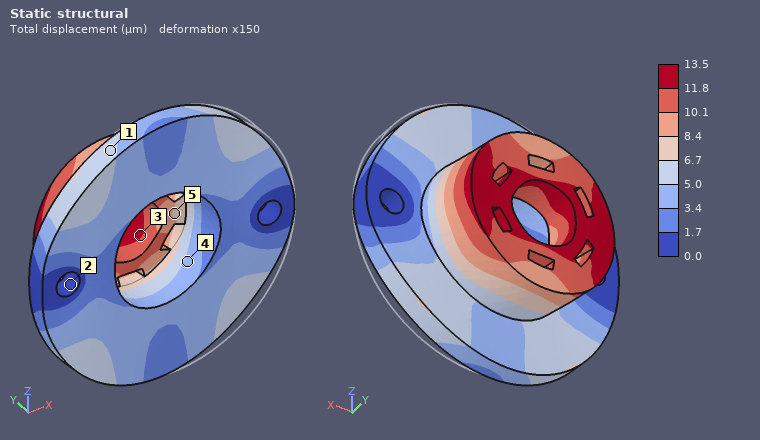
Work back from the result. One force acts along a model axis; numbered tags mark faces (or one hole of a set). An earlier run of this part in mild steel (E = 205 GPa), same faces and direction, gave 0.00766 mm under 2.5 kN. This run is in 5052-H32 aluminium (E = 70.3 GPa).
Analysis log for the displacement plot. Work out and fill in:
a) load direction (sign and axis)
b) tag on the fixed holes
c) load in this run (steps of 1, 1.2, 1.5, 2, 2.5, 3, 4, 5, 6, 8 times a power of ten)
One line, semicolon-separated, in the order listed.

-X; 2; 1.5 kN
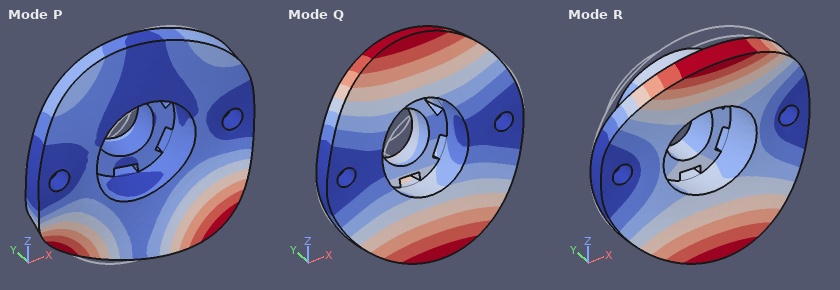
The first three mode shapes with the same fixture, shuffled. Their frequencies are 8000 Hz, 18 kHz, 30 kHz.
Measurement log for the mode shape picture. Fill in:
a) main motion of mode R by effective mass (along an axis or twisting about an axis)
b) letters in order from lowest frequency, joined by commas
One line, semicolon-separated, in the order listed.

along Y; Q, R, P
